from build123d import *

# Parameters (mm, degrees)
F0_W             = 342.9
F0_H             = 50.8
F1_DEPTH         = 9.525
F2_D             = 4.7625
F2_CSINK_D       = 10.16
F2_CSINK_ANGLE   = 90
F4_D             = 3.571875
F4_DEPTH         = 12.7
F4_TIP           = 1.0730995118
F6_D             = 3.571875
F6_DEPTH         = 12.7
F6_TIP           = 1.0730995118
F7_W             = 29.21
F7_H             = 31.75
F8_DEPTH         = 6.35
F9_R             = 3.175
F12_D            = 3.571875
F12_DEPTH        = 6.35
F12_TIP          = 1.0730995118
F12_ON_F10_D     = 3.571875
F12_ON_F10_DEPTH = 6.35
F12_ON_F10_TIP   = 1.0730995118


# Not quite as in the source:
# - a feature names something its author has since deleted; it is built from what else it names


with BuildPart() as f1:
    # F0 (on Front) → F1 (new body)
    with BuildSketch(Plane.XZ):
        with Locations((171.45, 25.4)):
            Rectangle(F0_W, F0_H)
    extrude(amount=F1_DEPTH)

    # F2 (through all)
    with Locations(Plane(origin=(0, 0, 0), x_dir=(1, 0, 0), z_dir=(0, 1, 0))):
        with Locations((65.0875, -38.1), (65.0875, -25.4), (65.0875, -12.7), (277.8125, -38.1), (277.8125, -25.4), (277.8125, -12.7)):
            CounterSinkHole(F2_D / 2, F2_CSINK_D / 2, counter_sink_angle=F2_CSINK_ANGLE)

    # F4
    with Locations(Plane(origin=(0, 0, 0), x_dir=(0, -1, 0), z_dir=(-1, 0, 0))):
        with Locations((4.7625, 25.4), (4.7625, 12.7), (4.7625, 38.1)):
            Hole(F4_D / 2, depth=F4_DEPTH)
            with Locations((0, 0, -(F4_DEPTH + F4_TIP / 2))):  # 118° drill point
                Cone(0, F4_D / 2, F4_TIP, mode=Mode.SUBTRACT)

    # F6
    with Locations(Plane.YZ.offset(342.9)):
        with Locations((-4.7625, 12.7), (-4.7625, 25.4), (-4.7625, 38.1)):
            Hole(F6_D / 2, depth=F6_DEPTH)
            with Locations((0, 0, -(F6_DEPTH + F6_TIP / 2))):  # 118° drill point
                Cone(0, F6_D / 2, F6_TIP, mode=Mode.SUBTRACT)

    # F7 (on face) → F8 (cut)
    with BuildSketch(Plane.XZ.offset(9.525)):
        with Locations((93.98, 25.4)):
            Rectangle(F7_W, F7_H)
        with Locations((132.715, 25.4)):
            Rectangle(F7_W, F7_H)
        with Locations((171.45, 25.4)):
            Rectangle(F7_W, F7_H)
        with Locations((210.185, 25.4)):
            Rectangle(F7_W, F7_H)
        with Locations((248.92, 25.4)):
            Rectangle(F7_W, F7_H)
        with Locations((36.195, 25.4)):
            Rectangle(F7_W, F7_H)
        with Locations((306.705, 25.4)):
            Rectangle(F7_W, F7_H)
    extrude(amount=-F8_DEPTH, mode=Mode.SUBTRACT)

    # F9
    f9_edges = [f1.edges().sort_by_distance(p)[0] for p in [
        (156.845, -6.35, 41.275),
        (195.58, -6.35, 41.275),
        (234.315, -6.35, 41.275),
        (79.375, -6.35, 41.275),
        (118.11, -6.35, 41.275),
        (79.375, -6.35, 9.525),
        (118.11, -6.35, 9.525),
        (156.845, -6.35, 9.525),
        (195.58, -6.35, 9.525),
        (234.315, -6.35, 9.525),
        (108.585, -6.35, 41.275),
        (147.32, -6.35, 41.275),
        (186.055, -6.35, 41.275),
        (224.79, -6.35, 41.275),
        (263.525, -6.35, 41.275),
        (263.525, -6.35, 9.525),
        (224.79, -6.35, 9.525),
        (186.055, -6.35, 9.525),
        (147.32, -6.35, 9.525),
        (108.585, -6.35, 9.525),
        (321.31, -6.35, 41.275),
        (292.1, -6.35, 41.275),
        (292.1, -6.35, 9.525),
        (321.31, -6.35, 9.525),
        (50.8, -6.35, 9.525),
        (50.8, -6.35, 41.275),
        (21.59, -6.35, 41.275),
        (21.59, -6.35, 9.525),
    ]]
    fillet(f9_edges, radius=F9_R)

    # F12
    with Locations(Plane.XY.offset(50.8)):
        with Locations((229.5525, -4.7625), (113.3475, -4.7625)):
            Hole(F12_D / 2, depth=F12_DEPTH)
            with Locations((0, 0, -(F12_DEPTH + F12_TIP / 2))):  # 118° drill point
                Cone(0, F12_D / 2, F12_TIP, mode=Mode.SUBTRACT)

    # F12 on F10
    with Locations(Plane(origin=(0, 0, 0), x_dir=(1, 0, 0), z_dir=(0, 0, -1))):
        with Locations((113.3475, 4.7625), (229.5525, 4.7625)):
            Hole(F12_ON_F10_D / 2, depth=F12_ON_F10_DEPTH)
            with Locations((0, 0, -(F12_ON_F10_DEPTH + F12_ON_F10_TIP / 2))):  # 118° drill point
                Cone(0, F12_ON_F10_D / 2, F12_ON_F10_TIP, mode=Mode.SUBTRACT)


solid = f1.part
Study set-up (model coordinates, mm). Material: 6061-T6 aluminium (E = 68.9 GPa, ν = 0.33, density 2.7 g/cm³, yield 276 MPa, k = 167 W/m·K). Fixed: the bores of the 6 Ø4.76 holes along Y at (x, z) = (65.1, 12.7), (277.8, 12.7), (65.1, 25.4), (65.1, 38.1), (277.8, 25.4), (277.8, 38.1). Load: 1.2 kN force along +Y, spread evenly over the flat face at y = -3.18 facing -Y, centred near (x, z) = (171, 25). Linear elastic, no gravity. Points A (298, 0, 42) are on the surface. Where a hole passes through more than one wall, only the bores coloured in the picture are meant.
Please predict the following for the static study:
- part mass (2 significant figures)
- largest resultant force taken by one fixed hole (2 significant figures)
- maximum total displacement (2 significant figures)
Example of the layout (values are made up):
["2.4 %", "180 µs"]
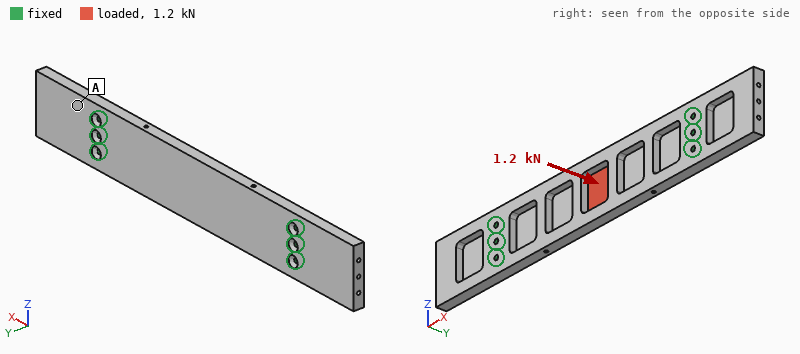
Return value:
["330 g", "520 N", "0.41 mm"]
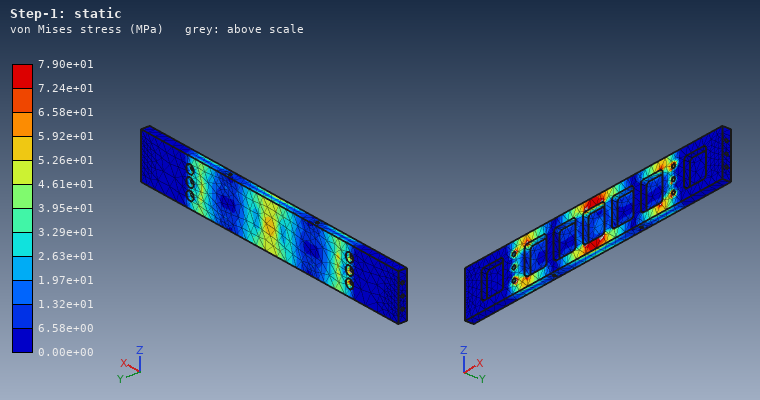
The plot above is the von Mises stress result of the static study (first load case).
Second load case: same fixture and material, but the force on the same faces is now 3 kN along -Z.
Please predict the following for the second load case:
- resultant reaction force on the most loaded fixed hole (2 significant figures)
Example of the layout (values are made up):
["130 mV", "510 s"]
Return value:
["2.5 kN"]
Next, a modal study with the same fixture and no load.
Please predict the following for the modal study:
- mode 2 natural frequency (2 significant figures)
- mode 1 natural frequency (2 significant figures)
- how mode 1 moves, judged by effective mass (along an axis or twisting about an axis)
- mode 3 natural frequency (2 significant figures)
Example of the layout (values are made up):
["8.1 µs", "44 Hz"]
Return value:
["1500 Hz", "1000 Hz", "along Y", "1500 Hz"]
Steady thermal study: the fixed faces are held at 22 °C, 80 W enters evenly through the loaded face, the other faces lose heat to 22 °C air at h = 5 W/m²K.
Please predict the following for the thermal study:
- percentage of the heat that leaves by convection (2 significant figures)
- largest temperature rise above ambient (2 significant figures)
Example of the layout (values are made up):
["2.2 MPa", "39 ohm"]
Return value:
["6.9 %", "83 K"]
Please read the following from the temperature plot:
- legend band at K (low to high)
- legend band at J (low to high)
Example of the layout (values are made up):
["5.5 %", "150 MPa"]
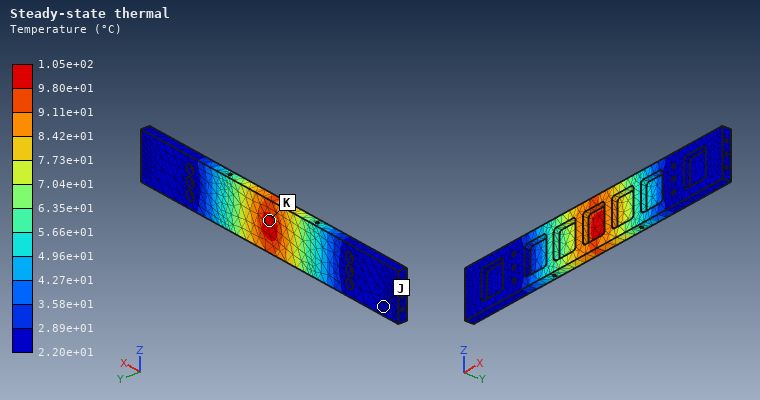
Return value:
["9.80e+01 to 1.05e+02 °C", "2.20e+01 to 2.89e+01 °C"]
